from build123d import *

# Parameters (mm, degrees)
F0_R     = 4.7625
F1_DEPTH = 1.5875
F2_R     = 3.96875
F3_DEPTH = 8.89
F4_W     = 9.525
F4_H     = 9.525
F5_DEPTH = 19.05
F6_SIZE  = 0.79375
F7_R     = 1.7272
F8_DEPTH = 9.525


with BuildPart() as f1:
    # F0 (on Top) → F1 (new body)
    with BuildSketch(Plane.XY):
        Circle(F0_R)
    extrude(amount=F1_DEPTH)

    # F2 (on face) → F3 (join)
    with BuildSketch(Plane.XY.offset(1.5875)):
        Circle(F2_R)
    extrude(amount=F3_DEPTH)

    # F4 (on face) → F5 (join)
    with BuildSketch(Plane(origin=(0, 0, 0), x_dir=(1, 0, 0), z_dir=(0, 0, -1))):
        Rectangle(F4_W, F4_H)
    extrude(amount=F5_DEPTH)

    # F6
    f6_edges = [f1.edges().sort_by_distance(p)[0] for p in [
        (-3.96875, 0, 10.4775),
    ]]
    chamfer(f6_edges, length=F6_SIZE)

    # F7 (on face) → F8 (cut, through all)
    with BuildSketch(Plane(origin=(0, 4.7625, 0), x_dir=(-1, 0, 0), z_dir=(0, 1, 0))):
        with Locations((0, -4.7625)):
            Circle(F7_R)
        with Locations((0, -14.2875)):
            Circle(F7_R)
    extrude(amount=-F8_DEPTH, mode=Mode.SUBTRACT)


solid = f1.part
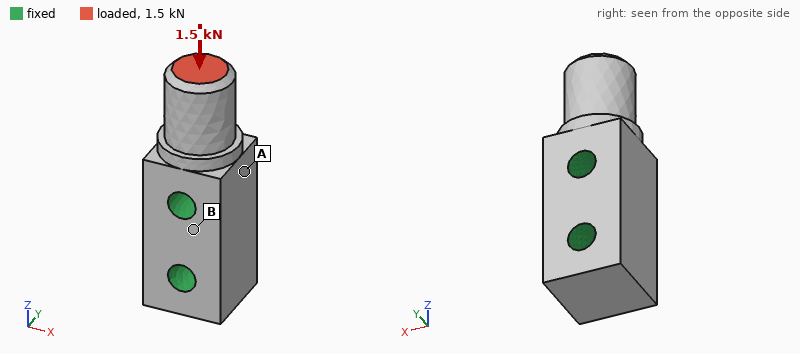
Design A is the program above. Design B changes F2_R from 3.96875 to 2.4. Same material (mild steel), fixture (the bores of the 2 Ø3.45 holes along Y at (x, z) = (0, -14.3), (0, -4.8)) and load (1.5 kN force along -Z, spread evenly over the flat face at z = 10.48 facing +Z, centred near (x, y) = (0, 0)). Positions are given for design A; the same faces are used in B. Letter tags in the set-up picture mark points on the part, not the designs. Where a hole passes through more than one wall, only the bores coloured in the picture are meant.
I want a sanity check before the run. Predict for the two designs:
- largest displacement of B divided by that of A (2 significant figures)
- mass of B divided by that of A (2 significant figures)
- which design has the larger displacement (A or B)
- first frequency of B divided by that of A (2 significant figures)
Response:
2.5
0.87
B
1.0
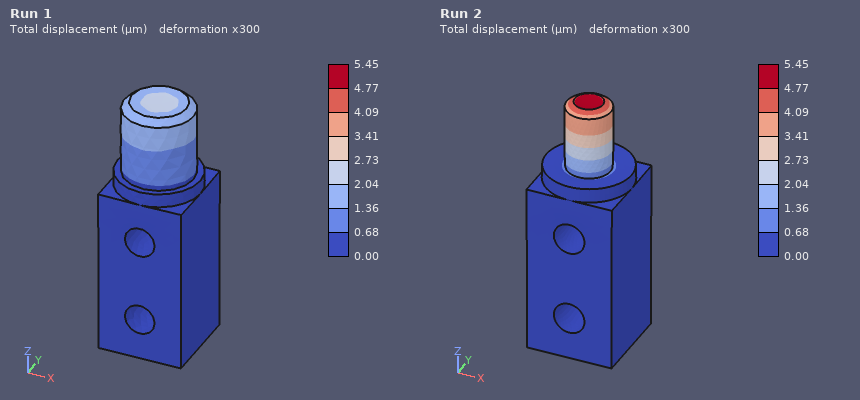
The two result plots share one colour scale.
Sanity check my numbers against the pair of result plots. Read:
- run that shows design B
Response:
Run 2
